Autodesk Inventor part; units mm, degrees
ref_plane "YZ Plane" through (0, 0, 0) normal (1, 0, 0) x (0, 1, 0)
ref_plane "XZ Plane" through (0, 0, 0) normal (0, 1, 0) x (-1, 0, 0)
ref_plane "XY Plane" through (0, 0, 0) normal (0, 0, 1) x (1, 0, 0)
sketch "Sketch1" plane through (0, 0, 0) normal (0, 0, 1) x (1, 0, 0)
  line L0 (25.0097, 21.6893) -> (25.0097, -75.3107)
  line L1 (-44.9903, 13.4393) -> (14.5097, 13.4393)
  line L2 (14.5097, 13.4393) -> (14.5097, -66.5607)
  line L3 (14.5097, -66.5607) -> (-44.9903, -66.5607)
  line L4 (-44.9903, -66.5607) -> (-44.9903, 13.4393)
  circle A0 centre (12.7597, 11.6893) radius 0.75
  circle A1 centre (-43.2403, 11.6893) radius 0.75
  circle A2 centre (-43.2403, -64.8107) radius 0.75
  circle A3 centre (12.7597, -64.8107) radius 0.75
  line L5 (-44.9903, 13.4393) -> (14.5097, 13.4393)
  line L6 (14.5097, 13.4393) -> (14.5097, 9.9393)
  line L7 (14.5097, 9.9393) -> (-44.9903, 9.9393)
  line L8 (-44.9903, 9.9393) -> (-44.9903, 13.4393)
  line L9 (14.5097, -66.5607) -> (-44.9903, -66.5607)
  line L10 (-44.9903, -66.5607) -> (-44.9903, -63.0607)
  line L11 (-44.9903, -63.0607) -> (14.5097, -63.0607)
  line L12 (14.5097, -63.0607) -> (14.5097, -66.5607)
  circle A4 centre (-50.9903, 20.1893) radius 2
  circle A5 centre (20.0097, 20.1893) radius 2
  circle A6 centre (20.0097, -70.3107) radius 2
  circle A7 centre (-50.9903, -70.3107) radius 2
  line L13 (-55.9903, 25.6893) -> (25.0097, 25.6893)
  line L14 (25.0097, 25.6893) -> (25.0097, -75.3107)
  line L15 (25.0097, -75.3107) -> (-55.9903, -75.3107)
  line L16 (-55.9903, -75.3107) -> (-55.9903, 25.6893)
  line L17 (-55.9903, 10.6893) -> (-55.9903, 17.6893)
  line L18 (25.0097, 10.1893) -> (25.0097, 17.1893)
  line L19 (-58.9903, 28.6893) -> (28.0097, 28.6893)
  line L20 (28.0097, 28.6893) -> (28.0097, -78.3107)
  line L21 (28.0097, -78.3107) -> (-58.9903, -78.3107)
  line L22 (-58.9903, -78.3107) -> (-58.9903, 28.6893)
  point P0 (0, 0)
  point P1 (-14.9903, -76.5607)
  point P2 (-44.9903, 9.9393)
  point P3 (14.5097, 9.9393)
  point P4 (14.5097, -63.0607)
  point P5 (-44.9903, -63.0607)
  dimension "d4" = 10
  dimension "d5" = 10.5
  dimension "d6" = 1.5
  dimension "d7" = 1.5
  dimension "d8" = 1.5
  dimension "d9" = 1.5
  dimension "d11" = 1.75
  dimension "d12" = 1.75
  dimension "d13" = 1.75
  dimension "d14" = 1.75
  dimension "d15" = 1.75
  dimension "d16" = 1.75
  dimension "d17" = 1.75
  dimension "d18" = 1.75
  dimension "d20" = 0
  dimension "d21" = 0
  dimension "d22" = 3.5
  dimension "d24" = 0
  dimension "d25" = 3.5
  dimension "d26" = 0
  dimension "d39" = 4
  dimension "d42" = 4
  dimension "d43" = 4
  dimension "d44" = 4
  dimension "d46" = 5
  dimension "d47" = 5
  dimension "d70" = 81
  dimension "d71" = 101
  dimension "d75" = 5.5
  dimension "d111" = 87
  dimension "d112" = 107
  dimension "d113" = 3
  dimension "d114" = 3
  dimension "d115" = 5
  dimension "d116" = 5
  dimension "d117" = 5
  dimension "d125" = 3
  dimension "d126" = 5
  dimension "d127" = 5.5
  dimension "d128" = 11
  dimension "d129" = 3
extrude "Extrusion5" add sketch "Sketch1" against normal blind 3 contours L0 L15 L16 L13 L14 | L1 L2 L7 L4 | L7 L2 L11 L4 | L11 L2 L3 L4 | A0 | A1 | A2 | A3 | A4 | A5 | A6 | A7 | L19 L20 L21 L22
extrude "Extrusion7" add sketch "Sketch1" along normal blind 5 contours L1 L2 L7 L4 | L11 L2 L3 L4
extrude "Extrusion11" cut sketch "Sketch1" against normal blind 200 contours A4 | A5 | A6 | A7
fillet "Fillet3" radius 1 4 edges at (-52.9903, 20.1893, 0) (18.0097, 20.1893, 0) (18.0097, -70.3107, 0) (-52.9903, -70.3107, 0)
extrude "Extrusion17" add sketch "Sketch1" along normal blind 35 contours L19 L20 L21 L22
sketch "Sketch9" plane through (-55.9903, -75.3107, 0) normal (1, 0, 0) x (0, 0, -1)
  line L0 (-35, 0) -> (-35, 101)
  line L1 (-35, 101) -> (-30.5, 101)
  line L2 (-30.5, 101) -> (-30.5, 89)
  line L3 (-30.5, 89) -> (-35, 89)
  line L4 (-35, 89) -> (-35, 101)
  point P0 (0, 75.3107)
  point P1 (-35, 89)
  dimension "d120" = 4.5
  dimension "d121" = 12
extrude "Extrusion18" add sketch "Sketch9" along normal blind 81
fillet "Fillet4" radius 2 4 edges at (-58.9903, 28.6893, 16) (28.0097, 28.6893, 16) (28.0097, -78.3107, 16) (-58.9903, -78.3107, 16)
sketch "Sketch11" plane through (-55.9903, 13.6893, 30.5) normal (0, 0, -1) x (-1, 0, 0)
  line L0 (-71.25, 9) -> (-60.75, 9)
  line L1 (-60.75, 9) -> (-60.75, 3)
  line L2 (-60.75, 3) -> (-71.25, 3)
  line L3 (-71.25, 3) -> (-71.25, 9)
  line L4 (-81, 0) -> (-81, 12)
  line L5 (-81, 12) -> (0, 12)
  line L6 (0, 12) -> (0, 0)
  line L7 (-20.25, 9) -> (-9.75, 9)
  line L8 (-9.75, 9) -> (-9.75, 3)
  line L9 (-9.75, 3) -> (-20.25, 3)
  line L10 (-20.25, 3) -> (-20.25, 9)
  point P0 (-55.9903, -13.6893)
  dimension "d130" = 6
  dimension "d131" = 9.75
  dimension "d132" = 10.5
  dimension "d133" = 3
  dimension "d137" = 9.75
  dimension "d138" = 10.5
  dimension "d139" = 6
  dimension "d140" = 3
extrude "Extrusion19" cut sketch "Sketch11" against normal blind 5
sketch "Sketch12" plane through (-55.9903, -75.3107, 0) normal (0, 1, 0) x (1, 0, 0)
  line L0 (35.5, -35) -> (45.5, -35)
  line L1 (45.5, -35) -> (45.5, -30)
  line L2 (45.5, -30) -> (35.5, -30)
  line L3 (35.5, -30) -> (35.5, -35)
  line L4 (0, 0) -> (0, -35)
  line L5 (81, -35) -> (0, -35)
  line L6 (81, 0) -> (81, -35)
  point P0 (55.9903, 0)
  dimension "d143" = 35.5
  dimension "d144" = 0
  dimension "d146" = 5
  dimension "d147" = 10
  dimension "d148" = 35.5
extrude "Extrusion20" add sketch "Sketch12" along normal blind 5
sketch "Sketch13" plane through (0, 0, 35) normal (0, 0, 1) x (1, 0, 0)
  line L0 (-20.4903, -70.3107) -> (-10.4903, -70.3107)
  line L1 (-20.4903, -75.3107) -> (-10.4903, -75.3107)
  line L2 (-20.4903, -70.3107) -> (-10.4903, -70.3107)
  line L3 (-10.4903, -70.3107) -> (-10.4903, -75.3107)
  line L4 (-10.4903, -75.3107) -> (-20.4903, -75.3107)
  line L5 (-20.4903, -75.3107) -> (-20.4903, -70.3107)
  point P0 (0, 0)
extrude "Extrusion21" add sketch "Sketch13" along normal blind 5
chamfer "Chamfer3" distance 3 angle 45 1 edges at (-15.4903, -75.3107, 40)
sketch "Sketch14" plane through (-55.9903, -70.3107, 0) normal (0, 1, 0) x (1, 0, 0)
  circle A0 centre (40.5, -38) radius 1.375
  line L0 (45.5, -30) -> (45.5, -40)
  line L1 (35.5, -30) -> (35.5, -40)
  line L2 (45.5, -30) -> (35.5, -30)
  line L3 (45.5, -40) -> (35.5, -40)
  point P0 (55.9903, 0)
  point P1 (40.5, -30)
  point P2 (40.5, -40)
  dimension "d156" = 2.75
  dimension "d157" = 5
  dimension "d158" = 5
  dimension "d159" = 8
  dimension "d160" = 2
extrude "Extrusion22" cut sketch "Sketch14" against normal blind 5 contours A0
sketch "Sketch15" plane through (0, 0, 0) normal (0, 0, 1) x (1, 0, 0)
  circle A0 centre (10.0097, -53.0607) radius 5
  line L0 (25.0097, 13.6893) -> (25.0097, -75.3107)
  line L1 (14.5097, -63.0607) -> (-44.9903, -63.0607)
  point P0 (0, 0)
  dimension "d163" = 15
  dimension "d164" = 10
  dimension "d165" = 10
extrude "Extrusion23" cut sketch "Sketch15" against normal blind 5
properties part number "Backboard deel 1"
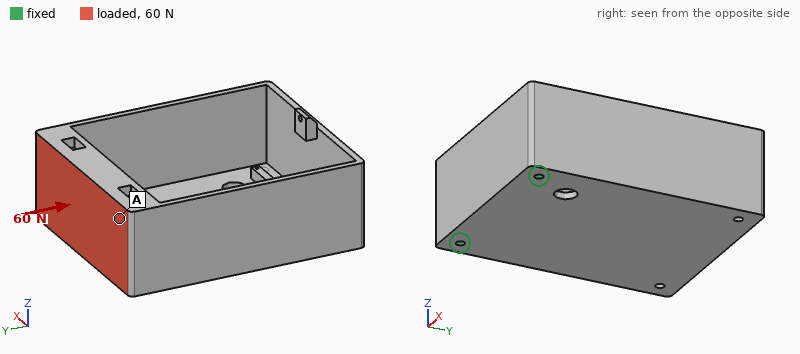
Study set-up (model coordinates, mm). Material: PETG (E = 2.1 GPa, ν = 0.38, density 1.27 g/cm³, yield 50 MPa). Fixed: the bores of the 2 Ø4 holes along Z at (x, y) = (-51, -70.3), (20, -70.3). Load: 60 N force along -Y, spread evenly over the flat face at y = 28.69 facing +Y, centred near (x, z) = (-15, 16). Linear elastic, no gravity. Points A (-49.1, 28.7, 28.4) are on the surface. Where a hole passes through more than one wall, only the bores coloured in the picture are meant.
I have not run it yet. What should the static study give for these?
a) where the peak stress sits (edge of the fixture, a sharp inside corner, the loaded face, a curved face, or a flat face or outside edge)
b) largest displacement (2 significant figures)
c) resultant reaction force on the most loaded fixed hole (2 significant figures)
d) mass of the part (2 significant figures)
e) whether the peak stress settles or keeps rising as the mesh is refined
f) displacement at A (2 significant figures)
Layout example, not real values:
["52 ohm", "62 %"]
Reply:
["edge of the fixture", "1.6 mm", "30 N", "93 g", "keeps rising", "1.6 mm"]
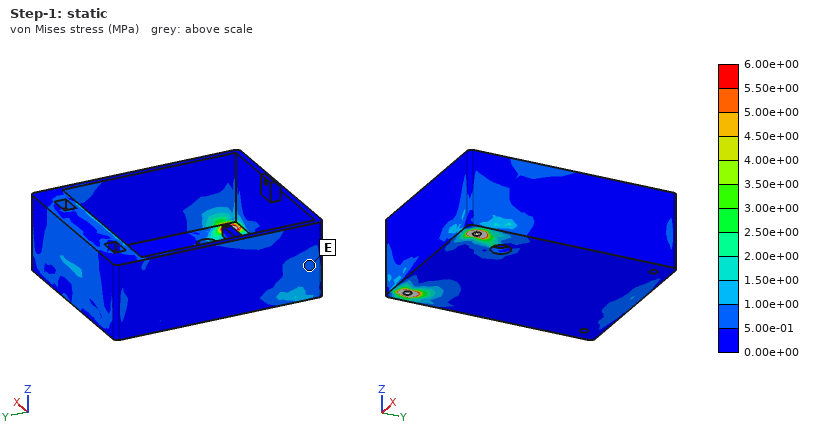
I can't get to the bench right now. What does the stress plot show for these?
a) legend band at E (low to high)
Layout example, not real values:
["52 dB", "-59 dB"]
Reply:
["5.00e-01 to 1.00e+00 MPa"]
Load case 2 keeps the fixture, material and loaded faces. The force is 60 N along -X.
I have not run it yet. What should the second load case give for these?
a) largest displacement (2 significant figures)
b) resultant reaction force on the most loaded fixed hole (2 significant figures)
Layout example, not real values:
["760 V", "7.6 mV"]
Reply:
["1.4 mm", "89 N"]
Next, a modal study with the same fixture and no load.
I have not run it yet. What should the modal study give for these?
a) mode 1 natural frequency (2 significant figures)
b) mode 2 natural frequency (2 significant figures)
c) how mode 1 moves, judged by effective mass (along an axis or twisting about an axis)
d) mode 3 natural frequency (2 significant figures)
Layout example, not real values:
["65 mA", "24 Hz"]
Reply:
["69 Hz", "150 Hz", "along Z", "550 Hz"]
